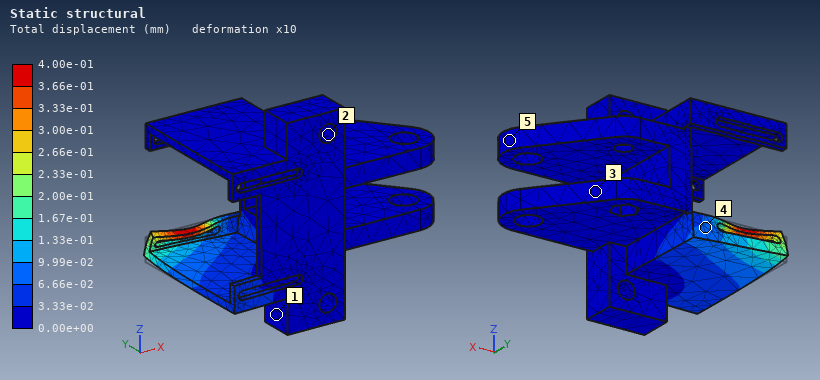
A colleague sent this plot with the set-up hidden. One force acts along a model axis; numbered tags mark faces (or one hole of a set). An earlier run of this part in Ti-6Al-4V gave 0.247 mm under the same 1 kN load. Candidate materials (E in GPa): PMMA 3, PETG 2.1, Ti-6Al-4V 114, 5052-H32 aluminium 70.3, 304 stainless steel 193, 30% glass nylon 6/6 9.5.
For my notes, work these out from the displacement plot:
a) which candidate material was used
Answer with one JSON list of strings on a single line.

["5052-H32 aluminium"]
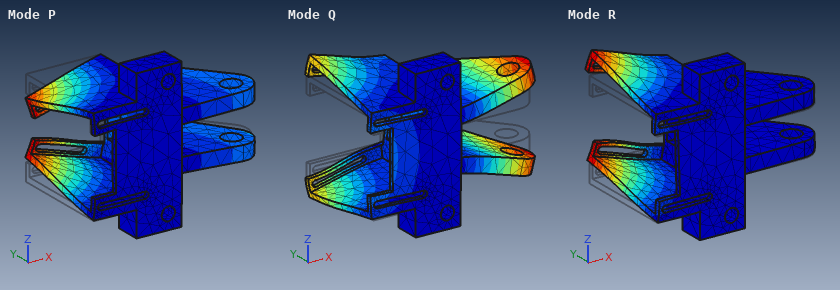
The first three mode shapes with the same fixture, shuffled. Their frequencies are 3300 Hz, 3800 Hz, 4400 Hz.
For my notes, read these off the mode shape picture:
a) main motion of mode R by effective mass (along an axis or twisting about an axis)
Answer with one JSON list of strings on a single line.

["along Z"]
